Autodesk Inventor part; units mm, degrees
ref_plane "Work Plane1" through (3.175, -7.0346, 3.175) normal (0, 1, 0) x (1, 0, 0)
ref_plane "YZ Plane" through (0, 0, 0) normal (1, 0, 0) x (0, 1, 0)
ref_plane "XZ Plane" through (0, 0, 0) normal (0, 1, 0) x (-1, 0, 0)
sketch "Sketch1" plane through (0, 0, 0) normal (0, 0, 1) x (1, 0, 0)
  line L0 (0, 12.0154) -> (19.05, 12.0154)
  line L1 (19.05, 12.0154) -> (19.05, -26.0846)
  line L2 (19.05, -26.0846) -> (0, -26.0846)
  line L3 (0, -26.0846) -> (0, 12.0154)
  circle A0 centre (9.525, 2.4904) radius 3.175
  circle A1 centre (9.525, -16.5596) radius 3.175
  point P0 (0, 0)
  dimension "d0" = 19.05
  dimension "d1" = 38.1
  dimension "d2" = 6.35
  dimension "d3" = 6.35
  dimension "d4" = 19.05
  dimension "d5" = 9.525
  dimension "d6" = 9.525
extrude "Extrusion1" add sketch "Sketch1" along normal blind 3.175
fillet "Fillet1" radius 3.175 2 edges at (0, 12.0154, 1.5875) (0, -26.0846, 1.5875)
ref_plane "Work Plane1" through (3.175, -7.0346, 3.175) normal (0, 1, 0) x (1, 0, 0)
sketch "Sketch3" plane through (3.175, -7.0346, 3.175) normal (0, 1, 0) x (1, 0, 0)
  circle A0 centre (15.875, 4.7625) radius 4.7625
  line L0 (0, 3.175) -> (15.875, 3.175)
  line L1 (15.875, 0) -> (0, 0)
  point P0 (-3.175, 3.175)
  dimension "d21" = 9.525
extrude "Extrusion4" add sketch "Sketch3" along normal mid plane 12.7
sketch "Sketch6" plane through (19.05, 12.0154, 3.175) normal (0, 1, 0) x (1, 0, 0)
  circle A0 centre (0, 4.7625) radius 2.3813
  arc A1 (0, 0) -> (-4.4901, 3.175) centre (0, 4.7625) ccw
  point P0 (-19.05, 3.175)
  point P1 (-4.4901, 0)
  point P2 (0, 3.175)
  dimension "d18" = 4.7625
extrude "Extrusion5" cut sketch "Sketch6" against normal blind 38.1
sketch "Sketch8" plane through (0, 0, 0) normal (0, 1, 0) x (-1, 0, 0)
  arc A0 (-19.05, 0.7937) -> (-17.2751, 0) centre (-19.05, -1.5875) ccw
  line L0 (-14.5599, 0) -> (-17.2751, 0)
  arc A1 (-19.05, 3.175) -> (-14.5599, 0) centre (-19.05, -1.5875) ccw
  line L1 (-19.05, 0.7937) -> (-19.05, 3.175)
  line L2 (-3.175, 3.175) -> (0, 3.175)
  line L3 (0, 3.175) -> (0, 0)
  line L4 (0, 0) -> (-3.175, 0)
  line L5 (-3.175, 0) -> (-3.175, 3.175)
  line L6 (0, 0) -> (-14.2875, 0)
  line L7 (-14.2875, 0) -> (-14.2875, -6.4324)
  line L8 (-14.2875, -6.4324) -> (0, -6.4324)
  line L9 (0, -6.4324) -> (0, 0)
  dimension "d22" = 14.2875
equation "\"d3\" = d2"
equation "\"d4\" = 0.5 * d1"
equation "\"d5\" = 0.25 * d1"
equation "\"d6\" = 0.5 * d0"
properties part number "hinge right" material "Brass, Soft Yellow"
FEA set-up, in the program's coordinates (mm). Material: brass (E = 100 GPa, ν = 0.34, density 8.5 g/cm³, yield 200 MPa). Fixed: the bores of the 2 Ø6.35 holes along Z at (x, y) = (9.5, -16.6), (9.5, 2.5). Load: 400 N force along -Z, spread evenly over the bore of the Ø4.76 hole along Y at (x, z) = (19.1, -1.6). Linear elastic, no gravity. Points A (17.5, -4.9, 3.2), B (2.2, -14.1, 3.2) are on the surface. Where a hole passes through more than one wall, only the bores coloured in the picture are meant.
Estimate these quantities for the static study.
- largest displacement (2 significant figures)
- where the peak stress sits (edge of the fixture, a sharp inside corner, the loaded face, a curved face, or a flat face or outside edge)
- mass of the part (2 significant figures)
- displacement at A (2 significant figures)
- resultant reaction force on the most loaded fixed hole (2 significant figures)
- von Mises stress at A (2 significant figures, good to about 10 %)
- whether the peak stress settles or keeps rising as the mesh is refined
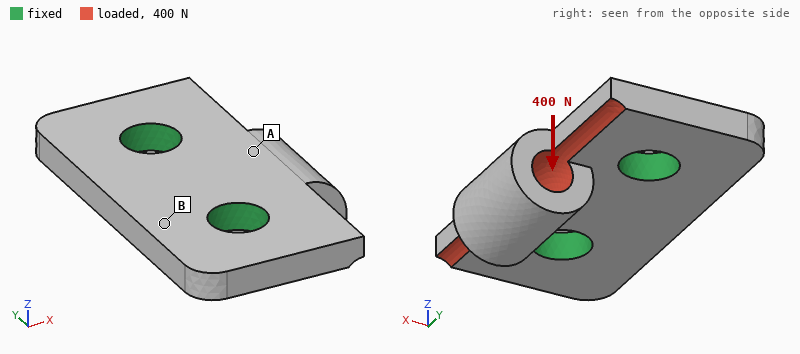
21 µm
edge of the fixture
22 g
8.5 µm
200 N
21 MPa
keeps rising
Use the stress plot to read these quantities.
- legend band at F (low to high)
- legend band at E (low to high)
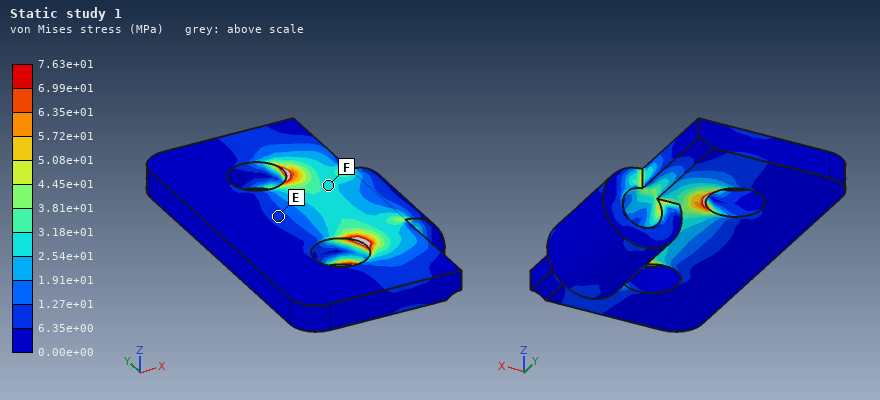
2.54e+01 to 3.18e+01 MPa
6.35e+00 to 1.27e+01 MPa
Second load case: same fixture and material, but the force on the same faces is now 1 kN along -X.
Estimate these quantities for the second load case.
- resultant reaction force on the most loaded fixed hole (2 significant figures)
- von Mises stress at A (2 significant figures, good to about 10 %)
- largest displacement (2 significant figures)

520 N
26 MPa
30 µm
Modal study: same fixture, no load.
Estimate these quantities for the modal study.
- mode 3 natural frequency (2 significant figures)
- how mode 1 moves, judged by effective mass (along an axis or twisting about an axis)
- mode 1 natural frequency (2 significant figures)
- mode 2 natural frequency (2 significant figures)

23 kHz
along Z
8800 Hz
22 kHz
